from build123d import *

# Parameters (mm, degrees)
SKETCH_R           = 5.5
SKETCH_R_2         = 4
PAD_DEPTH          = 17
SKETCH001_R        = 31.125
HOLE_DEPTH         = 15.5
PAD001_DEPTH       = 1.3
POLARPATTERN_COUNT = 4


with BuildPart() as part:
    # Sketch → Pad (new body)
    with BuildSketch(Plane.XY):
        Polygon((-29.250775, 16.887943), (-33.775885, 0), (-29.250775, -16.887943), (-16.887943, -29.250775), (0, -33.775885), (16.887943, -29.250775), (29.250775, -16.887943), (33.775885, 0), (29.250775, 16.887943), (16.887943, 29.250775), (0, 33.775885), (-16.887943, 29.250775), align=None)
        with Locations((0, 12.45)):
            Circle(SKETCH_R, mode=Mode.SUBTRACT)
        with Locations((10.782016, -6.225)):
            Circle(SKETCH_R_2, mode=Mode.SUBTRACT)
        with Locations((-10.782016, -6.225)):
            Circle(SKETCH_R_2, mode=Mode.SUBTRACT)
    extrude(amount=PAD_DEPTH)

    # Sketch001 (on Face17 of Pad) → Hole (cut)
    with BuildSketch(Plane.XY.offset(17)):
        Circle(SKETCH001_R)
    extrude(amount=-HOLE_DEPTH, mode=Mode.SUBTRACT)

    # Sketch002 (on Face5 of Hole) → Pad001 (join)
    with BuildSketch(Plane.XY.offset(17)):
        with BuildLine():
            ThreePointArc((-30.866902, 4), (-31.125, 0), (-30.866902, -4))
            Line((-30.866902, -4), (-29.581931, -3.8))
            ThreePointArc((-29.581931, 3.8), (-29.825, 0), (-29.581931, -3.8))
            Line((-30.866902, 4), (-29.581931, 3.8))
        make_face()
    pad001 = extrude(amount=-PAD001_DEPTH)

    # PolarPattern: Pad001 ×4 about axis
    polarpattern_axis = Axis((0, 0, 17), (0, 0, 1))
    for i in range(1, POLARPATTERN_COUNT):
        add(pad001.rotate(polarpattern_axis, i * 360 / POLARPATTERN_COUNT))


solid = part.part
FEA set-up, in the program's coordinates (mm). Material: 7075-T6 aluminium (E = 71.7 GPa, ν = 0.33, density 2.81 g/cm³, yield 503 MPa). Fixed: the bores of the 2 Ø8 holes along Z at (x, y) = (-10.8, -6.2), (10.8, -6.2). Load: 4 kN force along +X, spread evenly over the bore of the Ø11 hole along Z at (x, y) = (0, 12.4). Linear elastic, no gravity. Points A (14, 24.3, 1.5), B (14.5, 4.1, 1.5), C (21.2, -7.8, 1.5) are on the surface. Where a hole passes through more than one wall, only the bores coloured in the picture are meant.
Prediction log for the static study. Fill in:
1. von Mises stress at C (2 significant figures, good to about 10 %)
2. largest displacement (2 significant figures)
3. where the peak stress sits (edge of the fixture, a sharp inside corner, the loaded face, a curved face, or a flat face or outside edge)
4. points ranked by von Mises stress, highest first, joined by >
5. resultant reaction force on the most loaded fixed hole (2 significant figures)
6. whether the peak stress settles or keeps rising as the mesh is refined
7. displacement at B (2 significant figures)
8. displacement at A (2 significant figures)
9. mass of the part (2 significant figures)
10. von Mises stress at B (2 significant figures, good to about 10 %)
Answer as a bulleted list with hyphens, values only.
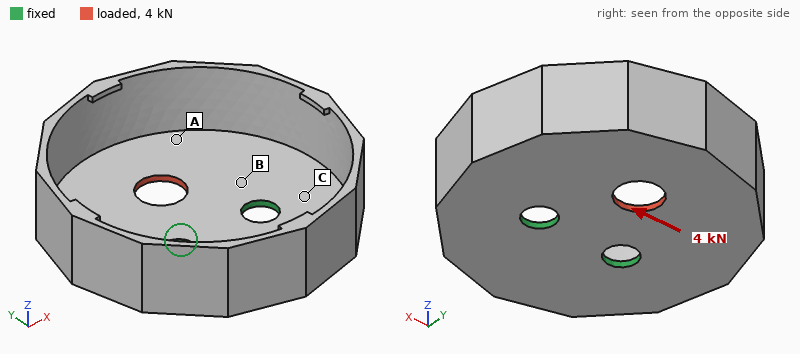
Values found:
- 41 MPa
- 99 µm
- edge of the fixture
- B > C > A
- 3.1 kN
- keeps rising
- 29 µm
- 78 µm
- 30 g
- 78 MPa
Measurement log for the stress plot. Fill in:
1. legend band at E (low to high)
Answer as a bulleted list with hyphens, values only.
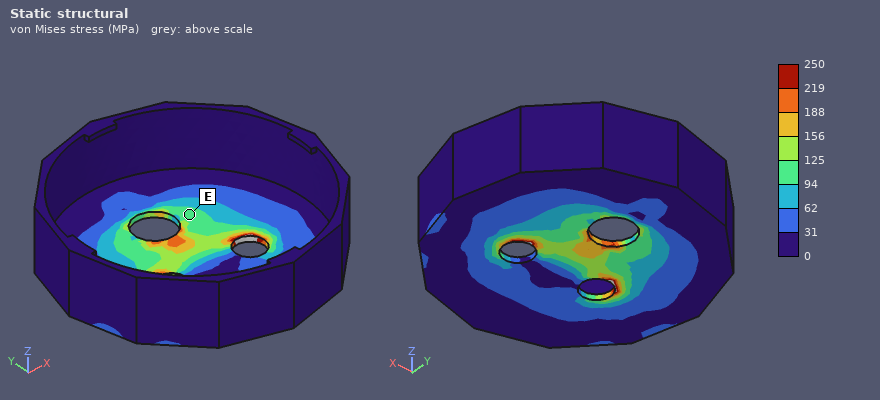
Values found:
- 94 to 125 MPa
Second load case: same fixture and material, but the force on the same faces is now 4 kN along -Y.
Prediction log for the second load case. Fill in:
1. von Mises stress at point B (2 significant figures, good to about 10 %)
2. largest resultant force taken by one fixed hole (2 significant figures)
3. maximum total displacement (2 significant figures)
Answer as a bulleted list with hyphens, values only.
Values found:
- 51 MPa
- 2.1 kN
- 33 µm
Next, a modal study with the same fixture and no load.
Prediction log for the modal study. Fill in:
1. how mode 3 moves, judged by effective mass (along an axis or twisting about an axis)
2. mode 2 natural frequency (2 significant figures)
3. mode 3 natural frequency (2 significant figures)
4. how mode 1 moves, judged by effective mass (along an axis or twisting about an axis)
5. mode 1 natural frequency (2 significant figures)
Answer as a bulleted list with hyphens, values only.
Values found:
- along Z
- 1700 Hz
- 2300 Hz
- along Z
- 850 Hz
